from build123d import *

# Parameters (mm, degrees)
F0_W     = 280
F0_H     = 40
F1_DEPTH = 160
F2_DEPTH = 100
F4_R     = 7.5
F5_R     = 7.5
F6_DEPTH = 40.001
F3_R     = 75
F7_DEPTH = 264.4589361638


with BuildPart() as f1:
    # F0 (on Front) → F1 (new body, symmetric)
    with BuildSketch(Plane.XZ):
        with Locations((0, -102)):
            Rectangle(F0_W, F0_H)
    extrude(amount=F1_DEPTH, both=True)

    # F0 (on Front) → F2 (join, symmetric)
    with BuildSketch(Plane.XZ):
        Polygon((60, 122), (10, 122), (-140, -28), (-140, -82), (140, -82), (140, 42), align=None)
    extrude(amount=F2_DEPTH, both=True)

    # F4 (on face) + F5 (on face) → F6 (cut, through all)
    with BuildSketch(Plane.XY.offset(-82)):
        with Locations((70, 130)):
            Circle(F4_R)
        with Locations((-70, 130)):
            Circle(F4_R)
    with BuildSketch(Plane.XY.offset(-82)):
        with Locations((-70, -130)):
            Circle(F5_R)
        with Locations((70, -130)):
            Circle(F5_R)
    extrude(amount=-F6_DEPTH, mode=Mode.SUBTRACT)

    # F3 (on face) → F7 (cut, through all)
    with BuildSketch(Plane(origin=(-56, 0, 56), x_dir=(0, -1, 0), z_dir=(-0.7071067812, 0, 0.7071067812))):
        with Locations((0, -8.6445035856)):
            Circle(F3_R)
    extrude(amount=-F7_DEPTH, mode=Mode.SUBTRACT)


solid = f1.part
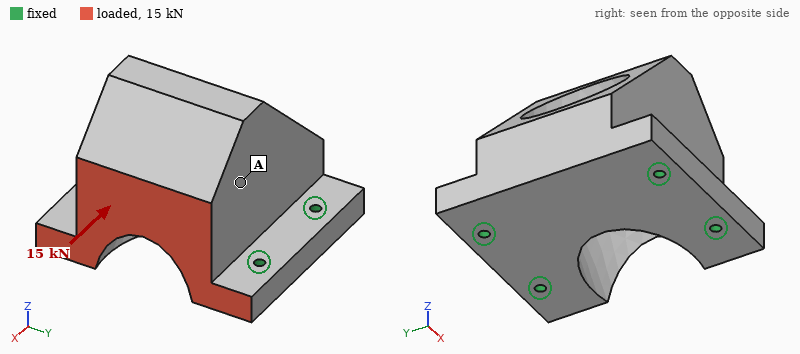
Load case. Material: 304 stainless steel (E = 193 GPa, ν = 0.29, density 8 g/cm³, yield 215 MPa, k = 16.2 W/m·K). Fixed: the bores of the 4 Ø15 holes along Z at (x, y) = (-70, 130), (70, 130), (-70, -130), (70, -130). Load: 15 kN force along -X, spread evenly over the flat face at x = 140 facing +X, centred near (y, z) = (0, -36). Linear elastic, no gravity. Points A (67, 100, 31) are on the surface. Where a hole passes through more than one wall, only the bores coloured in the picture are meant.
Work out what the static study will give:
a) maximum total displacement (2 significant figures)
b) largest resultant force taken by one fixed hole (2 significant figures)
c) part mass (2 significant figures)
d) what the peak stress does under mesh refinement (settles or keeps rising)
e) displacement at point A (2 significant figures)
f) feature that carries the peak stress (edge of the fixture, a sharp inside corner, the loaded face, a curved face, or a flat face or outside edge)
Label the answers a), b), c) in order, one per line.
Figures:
a) 6.1 µm
b) 5.4 kN
c) 64 kg
d) keeps rising
e) 4.3 µm
f) edge of the fixture
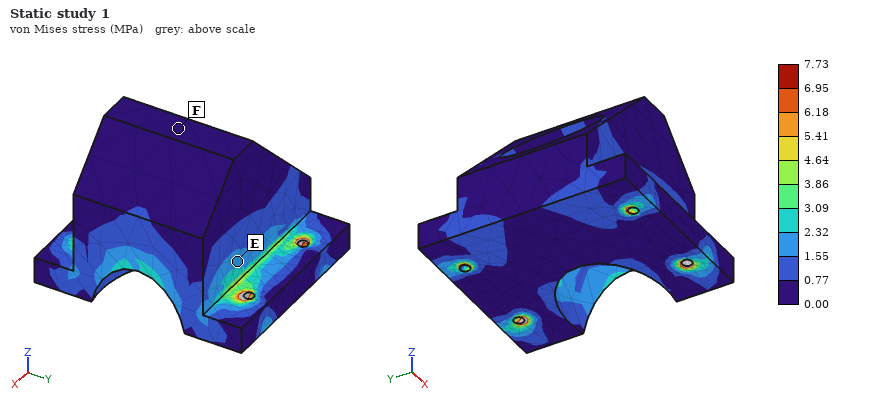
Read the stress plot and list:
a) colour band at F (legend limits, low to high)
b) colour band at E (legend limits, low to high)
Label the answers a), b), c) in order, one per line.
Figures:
a) 0.00 to 0.77 MPa
b) 1.55 to 2.32 MPa
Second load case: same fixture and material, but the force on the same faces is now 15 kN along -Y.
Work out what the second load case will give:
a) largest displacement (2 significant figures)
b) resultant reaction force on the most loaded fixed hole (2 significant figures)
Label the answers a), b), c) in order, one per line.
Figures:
a) 6.6 µm
b) 8.4 kN
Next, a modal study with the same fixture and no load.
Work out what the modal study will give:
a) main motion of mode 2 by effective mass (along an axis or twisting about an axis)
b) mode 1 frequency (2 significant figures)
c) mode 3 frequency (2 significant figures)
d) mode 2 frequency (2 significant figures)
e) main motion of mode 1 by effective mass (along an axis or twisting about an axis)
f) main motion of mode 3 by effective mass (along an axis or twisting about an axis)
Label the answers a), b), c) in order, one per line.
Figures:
a) along Y
b) 1100 Hz
c) 2000 Hz
d) 1400 Hz
e) along X
f) along Z
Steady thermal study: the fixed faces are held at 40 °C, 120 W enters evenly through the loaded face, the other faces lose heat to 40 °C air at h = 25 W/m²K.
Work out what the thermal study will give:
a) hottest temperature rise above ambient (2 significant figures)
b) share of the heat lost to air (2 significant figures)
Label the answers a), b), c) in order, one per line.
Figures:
a) 40 K
b) 69 %
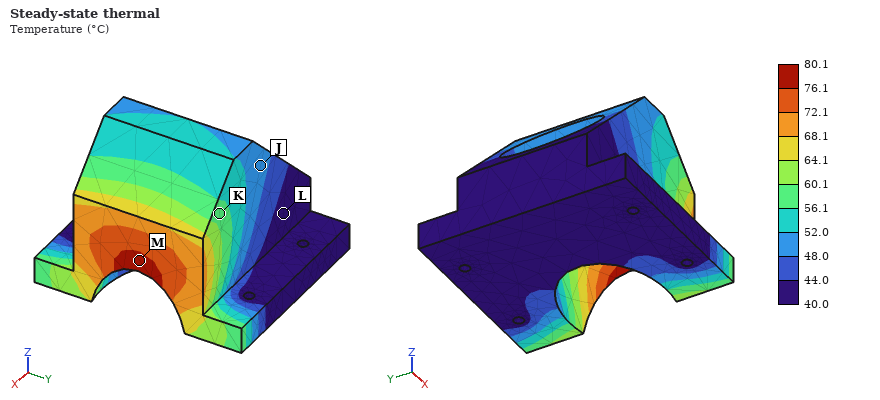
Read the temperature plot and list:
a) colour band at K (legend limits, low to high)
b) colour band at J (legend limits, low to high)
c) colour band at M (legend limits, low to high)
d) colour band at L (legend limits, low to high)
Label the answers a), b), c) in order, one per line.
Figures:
a) 56.1 to 60.1 °C
b) 48.0 to 52.0 °C
c) 76.1 to 80.1 °C
d) 40.0 to 44.0 °C
